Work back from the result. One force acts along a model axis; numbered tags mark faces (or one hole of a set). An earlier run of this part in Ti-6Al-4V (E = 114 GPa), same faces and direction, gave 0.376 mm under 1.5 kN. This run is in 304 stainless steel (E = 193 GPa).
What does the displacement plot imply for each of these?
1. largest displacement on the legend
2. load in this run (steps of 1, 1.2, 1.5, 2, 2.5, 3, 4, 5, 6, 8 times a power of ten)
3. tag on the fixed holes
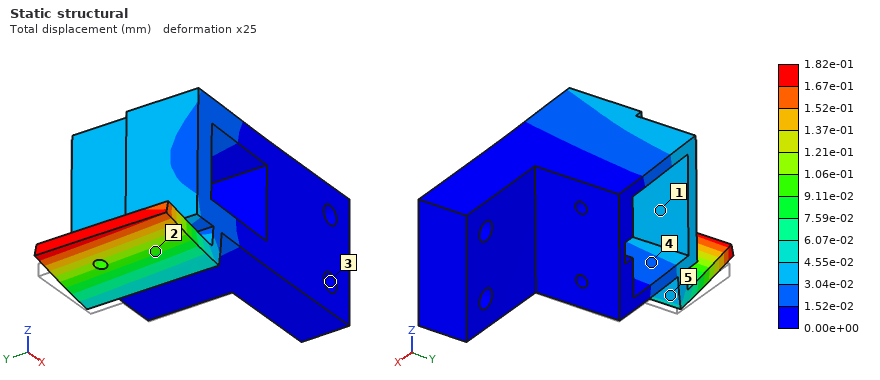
1.82e-01 mm
1.2 kN
3
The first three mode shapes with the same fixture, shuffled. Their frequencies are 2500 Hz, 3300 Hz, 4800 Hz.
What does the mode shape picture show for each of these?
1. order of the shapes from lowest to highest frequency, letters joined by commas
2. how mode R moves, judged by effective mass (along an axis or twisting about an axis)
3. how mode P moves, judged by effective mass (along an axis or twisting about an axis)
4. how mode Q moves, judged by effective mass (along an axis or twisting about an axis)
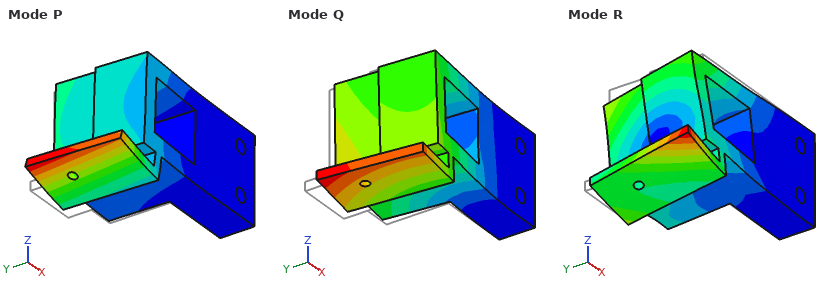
Q, P, R
twisting about X
along Z
along Y
